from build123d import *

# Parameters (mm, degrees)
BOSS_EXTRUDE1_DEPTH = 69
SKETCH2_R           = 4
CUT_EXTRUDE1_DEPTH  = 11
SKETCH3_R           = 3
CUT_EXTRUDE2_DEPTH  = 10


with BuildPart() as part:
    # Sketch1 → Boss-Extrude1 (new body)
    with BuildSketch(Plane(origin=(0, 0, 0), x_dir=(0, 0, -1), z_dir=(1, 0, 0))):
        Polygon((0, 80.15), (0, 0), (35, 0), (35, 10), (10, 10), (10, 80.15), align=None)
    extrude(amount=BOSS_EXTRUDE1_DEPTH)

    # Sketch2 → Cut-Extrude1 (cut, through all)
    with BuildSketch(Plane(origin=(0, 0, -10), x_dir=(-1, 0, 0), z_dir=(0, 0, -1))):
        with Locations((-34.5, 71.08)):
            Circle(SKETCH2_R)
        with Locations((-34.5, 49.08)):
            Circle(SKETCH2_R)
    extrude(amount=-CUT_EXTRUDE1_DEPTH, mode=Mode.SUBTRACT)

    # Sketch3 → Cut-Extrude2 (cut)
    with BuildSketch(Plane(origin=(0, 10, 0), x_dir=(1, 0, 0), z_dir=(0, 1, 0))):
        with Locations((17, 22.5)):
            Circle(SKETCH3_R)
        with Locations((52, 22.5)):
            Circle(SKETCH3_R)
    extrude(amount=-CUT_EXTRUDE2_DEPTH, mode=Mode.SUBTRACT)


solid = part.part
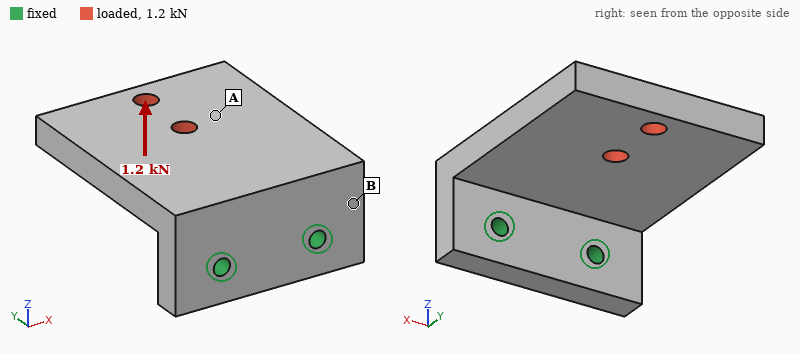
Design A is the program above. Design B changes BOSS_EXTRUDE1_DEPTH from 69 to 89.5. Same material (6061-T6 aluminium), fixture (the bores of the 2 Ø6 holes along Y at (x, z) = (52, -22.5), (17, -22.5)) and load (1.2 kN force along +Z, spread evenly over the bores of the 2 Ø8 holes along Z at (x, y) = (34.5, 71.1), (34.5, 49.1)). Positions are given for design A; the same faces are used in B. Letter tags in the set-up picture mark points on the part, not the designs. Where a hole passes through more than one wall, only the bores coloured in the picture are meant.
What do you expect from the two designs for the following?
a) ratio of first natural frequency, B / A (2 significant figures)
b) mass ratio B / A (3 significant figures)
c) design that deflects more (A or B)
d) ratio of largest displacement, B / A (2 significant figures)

0.94
1.30
A
0.86
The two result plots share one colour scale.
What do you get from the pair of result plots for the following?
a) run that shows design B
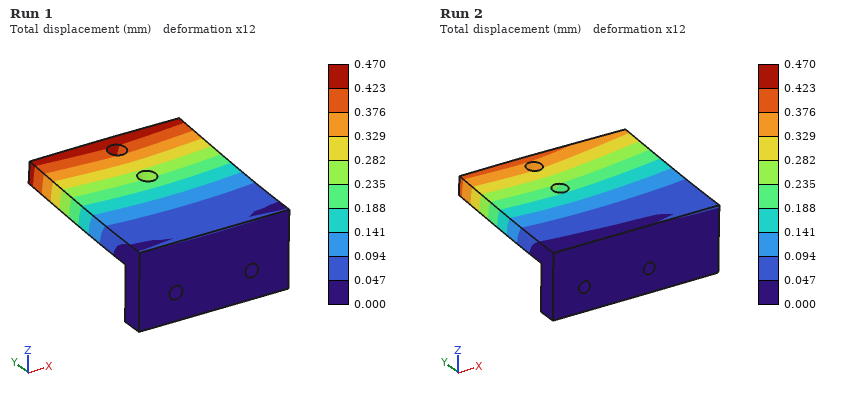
Run 2
